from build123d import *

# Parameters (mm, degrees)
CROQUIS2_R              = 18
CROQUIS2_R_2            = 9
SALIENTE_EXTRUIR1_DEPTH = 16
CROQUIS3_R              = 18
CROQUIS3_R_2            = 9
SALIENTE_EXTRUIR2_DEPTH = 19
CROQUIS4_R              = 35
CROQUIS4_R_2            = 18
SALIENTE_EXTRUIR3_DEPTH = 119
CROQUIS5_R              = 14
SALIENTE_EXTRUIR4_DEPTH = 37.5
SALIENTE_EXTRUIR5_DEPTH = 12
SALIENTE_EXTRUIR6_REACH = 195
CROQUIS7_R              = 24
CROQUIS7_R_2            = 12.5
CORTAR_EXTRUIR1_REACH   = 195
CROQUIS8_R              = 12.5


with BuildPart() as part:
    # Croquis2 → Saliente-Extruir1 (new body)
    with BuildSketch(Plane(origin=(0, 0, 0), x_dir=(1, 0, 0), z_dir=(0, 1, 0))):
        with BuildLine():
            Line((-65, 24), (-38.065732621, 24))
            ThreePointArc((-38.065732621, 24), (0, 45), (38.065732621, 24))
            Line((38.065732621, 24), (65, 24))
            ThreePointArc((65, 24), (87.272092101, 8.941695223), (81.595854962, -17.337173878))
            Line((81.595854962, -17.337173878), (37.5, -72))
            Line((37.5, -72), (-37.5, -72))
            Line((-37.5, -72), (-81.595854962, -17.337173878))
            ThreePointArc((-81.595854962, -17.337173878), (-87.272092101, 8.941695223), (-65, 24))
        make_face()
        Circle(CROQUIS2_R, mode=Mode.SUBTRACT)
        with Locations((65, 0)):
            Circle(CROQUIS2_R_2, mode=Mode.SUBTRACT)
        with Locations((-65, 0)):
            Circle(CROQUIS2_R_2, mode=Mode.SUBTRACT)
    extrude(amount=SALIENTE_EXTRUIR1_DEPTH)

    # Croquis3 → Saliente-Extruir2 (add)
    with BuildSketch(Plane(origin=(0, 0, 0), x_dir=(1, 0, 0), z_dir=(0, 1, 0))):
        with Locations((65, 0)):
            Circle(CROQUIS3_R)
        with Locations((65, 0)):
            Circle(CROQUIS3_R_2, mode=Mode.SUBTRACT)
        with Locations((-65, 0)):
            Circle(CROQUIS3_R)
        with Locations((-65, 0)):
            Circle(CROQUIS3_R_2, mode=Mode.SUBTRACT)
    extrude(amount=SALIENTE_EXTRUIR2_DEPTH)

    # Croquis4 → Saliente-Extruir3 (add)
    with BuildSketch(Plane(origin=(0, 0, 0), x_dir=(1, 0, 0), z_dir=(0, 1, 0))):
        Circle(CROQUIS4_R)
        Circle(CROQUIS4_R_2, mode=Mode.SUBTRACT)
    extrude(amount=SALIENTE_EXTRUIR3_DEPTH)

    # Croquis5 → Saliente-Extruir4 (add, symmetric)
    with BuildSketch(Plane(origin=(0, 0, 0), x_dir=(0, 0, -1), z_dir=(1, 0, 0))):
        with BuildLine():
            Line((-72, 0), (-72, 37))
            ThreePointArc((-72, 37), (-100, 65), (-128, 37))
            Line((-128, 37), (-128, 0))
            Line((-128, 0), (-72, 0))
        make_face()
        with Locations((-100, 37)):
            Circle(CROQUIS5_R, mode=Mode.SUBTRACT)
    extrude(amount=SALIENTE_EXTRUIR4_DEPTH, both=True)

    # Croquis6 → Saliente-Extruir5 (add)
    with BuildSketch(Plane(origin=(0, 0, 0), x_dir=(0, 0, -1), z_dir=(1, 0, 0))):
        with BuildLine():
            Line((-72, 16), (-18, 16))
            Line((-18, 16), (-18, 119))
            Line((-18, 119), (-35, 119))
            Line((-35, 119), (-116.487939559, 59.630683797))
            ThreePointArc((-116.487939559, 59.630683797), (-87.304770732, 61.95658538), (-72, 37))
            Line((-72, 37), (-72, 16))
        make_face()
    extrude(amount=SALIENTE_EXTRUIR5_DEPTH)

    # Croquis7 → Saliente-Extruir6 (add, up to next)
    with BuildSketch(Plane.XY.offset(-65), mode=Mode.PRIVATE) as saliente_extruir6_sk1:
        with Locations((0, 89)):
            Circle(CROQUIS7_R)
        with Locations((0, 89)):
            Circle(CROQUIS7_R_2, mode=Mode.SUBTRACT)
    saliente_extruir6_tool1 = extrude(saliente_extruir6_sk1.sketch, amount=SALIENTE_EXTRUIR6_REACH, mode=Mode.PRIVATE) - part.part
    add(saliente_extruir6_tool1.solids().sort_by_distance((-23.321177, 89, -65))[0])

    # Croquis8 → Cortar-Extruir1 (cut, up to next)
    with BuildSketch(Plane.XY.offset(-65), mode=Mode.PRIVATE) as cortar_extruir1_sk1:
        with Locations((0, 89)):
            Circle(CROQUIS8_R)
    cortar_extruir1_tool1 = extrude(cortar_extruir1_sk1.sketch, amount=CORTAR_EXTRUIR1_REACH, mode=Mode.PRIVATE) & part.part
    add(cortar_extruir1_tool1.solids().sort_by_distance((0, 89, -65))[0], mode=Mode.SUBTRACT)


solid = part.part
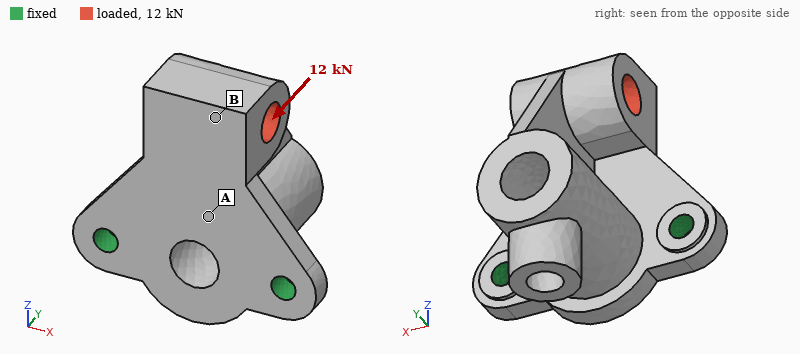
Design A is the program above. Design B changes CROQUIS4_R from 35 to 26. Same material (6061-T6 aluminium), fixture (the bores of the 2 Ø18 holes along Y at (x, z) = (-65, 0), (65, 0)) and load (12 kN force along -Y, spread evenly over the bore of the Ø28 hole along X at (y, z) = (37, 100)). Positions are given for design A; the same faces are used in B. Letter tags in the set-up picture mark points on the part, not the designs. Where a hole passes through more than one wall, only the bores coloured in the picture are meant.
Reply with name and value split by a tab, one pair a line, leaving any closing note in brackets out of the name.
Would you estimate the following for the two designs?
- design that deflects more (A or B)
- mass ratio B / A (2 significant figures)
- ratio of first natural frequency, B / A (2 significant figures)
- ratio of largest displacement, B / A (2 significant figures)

design that deflects more	B
mass ratio B / A	0.81
ratio of first natural frequency, B / A	0.99
ratio of largest displacement, B / A	1.2
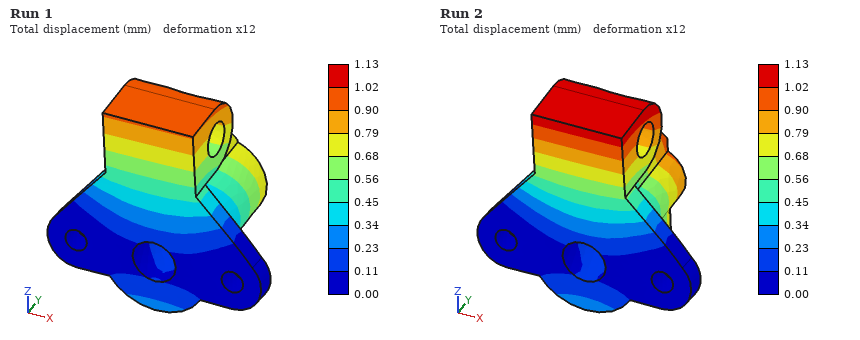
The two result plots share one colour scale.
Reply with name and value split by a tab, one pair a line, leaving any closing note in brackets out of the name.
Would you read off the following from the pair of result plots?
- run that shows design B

run that shows design B	Run 2
